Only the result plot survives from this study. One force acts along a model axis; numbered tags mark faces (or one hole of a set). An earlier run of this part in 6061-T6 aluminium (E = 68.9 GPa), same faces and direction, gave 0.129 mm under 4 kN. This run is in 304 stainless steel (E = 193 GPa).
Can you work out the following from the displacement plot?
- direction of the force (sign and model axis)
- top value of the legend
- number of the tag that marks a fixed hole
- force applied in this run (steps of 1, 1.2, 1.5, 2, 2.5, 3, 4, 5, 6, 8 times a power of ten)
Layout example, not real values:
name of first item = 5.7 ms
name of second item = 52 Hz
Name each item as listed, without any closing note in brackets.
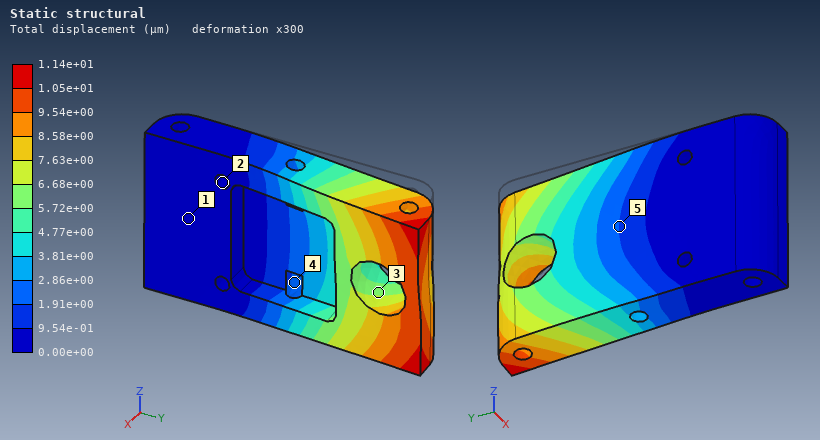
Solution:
direction of the force = -Z
top value of the legend = 1.14e+01 µm
number of the tag that marks a fixed hole = 2
force applied in this run = 1 kN
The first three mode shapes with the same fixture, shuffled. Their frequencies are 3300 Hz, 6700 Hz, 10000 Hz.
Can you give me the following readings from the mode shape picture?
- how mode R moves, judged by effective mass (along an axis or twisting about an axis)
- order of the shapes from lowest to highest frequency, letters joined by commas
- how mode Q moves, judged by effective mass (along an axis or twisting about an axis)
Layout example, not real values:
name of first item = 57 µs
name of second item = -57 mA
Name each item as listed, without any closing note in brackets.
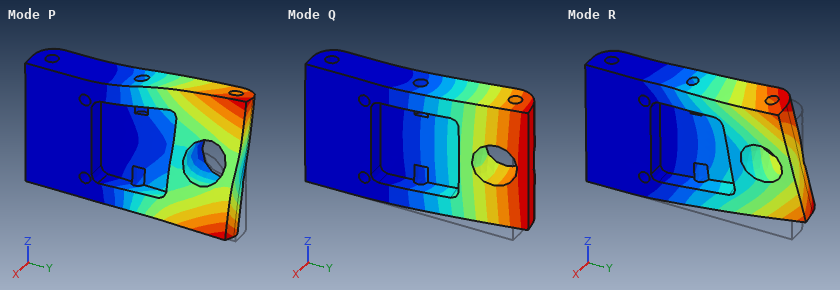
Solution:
how mode R moves, judged by effective mass = along Z
order of the shapes from lowest to highest frequency, letters joined by commas = Q, P, R
how mode Q moves, judged by effective mass = along X
